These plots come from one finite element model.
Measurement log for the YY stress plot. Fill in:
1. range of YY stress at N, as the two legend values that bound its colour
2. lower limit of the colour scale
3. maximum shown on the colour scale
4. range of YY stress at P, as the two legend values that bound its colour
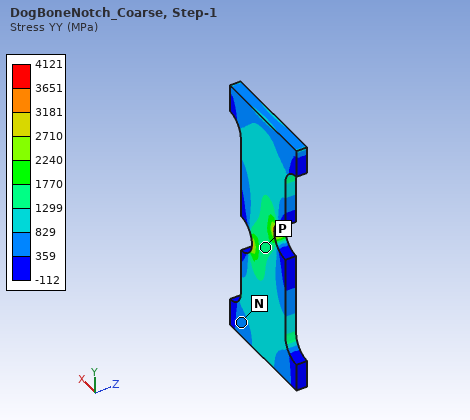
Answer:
359 to 829 MPa
-112 MPa
4121 MPa
1299 to 1770 MPa
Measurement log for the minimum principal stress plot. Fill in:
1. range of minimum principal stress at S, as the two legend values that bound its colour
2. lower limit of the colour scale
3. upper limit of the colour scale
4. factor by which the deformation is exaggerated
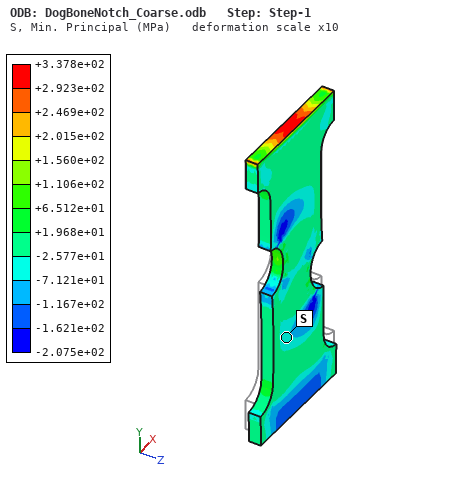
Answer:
-7.121e+01 to -2.577e+01 MPa
-2.075e+02 MPa
+3.378e+02 MPa
10
